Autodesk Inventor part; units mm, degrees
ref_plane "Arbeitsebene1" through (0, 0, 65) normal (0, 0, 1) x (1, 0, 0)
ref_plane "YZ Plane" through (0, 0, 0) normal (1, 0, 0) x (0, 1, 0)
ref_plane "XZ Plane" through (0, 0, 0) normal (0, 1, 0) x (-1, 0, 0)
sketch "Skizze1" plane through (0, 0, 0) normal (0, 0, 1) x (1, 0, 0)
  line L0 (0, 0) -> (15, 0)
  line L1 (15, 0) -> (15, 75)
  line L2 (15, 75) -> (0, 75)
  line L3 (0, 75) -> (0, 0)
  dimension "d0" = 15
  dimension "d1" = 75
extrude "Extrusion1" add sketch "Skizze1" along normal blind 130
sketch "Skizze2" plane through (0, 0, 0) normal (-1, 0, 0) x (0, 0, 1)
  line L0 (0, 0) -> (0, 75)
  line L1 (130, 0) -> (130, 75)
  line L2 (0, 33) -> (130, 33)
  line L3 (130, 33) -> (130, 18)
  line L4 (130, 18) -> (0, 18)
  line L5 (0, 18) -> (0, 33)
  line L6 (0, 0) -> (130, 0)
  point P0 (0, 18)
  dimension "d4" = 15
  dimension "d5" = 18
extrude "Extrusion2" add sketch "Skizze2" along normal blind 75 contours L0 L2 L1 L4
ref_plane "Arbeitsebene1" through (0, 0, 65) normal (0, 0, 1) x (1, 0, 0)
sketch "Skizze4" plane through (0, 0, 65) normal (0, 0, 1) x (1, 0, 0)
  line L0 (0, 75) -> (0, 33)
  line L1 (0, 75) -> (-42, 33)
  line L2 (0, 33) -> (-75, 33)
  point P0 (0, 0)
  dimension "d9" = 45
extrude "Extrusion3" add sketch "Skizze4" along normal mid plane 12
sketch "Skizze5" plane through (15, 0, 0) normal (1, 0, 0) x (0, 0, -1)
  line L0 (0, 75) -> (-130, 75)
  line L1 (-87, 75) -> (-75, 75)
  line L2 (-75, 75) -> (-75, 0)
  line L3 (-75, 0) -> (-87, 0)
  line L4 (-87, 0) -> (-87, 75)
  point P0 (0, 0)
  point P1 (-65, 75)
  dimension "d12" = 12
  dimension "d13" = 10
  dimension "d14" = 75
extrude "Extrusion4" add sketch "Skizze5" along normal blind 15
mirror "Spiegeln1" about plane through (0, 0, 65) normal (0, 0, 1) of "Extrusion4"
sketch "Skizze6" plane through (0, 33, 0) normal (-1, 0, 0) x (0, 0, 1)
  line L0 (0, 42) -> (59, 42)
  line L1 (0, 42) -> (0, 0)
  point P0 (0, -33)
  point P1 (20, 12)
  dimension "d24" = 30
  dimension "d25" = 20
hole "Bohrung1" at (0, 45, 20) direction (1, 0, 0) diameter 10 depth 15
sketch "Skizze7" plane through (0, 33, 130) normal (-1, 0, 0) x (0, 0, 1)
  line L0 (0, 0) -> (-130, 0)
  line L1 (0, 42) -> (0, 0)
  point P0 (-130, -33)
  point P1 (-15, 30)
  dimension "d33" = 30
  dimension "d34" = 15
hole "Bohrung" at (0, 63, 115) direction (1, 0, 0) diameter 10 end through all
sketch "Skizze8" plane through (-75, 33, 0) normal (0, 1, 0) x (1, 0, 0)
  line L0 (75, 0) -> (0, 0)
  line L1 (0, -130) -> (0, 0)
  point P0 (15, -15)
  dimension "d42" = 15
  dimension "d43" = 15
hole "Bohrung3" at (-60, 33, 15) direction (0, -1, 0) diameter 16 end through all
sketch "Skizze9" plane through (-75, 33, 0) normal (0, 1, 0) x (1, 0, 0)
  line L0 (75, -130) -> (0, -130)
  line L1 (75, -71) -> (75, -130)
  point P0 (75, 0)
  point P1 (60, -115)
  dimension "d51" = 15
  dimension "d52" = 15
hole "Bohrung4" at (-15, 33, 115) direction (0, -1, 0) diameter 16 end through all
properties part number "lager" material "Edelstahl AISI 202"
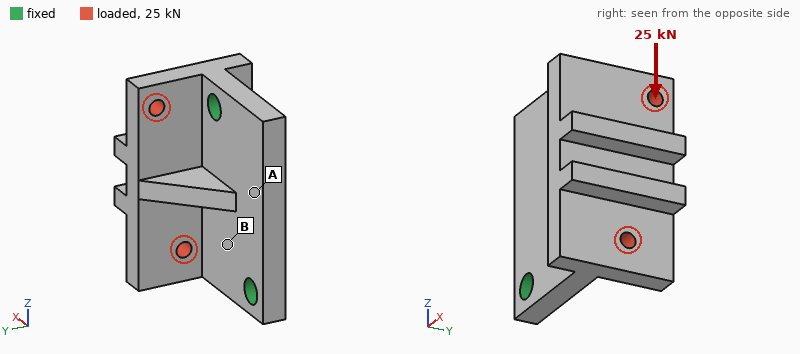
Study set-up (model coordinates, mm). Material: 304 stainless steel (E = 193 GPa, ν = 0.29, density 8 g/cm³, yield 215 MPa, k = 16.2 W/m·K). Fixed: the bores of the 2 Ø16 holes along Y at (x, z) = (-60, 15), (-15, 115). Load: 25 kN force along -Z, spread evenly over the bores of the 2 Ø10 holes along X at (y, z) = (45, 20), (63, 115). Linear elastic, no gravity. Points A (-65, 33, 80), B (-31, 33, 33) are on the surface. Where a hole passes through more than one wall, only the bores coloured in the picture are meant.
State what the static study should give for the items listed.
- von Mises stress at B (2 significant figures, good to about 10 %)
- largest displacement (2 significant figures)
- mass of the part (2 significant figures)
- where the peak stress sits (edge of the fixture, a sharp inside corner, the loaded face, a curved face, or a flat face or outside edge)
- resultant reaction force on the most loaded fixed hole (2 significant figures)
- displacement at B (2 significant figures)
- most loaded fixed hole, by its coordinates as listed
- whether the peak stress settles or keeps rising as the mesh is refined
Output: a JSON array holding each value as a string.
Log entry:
["46 MPa", "0.13 mm", "2.6 kg", "edge of the fixture", "21 kN", "0.023 mm", "(-15, 115)", "keeps rising"]
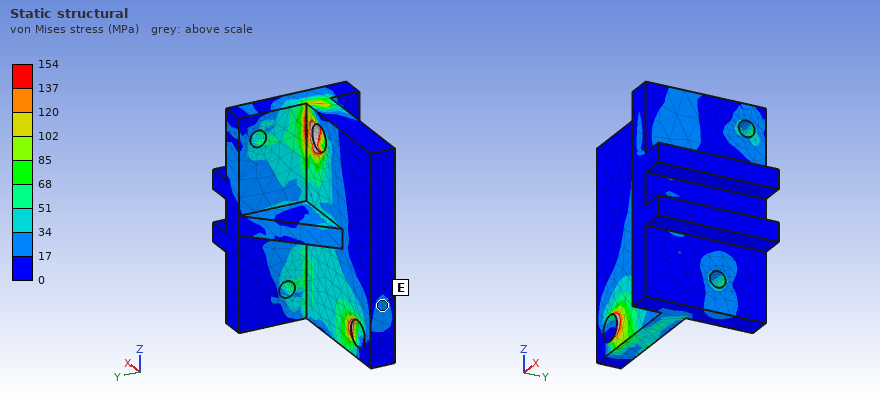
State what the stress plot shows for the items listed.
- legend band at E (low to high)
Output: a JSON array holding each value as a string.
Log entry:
["17 to 34 MPa"]
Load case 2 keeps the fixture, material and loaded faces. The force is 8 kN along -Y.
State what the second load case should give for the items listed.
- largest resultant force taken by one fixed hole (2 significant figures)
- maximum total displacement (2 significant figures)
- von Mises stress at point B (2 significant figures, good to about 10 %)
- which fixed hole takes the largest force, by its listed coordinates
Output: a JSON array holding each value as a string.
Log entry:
["5.5 kN", "83 µm", "24 MPa", "(-15, 115)"]
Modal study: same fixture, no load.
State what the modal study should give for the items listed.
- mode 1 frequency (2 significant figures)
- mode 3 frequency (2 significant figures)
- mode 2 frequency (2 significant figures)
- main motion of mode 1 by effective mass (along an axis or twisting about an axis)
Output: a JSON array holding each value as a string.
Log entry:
["1500 Hz", "4500 Hz", "3600 Hz", "along Y"]
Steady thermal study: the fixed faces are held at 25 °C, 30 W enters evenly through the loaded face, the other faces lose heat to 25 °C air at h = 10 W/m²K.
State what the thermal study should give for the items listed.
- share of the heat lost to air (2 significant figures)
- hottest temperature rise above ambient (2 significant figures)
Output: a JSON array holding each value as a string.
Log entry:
["37 %", "67 K"]
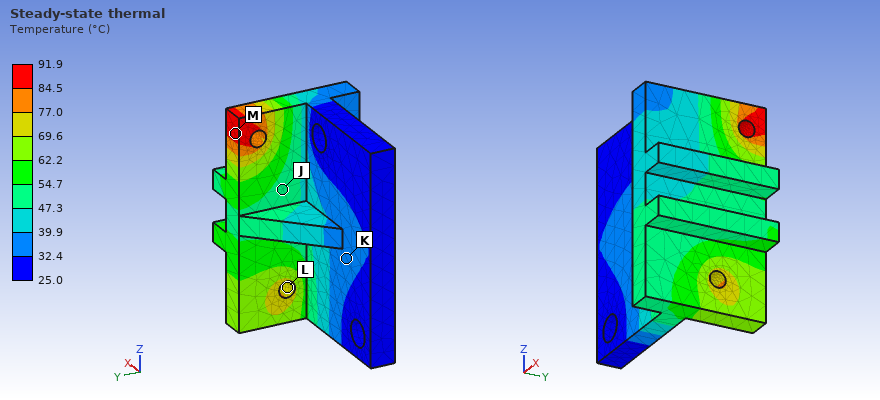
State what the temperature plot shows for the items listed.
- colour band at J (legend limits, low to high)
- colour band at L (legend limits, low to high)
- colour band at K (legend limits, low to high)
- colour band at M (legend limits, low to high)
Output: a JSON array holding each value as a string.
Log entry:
["47.3 to 54.7 °C", "69.6 to 77.0 °C", "32.4 to 39.9 °C", "84.5 to 91.9 °C"]
